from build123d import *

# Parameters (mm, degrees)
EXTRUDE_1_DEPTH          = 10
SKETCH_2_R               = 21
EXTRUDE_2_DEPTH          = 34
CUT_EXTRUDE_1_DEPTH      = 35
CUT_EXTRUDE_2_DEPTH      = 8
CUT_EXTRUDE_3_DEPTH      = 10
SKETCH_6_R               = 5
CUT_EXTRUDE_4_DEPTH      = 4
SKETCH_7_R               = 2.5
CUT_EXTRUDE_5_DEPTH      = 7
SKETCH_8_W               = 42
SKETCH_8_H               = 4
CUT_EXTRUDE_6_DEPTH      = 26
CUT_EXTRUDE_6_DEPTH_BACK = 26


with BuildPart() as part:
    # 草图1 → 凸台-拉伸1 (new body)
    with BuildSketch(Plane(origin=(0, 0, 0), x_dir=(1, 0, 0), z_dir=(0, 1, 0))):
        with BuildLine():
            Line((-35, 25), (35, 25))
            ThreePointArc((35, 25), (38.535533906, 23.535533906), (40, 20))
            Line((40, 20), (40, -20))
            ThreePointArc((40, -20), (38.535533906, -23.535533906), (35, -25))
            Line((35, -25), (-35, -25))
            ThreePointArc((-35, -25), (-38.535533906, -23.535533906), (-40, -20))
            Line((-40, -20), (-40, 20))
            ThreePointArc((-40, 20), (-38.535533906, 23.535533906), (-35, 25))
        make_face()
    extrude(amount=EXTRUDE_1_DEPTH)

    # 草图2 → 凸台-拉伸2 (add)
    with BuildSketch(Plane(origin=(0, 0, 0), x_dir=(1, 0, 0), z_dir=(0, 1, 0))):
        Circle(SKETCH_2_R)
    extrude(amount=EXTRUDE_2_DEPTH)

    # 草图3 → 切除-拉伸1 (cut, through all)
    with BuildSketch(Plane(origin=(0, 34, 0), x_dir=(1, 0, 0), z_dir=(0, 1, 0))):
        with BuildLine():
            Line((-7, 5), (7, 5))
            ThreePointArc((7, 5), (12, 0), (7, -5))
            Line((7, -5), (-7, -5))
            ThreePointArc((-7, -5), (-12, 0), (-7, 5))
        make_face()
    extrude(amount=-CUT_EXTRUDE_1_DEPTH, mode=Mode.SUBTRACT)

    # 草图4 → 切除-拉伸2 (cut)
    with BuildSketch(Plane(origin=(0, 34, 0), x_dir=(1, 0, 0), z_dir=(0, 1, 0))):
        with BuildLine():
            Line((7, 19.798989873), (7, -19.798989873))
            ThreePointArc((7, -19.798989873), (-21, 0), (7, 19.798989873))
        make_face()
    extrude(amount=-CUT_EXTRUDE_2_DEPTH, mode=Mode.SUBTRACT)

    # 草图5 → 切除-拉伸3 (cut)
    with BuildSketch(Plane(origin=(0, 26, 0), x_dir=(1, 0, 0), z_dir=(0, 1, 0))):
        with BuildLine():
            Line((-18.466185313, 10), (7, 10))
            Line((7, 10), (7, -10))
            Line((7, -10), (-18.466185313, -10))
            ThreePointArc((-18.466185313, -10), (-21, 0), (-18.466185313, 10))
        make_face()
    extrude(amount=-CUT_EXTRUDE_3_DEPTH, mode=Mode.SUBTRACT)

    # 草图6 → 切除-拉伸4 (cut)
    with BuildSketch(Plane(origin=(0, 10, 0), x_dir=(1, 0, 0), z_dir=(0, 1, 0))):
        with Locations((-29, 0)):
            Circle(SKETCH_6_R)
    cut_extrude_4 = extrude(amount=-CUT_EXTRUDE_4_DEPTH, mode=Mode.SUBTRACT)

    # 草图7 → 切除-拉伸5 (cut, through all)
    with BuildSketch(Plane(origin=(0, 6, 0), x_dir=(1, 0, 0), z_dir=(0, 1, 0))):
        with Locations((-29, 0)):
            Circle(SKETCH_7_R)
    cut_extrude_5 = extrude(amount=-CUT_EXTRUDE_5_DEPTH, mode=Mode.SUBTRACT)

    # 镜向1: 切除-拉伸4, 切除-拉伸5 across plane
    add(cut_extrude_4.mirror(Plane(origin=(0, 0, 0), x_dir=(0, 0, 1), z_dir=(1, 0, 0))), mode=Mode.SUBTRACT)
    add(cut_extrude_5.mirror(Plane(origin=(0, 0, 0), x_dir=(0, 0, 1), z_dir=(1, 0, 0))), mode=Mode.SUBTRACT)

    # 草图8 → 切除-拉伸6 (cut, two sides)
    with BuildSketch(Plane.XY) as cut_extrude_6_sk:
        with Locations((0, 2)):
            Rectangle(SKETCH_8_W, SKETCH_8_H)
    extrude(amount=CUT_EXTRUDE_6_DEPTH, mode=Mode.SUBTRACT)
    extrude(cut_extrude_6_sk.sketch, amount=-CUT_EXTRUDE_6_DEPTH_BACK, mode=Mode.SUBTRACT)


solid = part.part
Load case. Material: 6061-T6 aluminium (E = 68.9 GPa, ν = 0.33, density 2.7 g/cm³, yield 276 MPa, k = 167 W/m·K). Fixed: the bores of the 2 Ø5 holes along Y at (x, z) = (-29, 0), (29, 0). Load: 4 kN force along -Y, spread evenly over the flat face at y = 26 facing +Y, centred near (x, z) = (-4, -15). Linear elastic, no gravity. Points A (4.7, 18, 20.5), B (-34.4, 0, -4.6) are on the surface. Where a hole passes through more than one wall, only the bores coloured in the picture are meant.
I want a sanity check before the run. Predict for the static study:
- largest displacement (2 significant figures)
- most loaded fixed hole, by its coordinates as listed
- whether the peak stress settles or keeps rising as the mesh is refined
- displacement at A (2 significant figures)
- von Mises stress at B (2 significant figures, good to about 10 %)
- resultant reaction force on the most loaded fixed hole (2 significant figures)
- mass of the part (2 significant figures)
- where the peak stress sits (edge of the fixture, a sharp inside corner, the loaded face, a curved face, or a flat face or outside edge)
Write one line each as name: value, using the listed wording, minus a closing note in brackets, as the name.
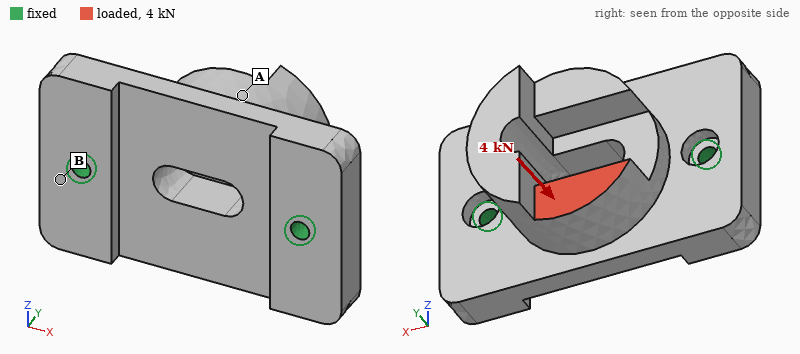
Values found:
largest displacement: 0.16 mm
most loaded fixed hole, by its coordinates as listed: (-29, 0)
whether the peak stress settles or keeps rising as the mesh is refined: keeps rising
displacement at A: 0.081 mm
von Mises stress at B: 55 MPa
resultant reaction force on the most loaded fixed hole: 3.1 kN
mass of the part: 130 g
where the peak stress sits: edge of the fixture
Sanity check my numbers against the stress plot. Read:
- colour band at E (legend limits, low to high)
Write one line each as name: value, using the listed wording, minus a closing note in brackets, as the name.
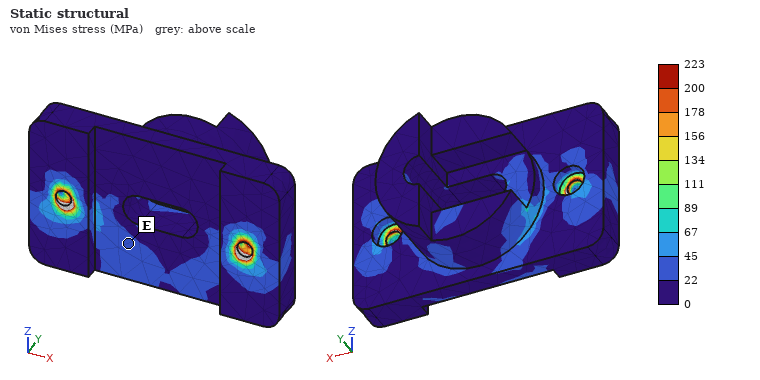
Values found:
colour band at E: 22 to 45 MPa
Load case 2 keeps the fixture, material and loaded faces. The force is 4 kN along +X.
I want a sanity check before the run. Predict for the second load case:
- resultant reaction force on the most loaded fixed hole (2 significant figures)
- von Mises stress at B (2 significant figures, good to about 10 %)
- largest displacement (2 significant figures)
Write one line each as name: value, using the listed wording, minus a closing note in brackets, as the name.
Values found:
resultant reaction force on the most loaded fixed hole: 2.9 kN
von Mises stress at B: 18 MPa
largest displacement: 41 µm
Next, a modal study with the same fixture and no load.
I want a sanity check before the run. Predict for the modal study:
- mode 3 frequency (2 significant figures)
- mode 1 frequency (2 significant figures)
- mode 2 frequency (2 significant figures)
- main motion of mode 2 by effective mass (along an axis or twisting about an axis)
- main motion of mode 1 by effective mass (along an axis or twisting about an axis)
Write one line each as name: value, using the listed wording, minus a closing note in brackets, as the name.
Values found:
mode 3 frequency: 9300 Hz
mode 1 frequency: 3300 Hz
mode 2 frequency: 8300 Hz
main motion of mode 2 by effective mass: along Y
main motion of mode 1 by effective mass: along Z
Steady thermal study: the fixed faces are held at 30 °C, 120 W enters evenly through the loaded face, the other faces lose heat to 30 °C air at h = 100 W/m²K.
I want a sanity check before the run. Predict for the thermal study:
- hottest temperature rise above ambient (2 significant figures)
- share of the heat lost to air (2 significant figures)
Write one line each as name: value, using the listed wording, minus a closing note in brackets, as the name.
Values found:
hottest temperature rise above ambient: 74 K
share of the heat lost to air: 22 %
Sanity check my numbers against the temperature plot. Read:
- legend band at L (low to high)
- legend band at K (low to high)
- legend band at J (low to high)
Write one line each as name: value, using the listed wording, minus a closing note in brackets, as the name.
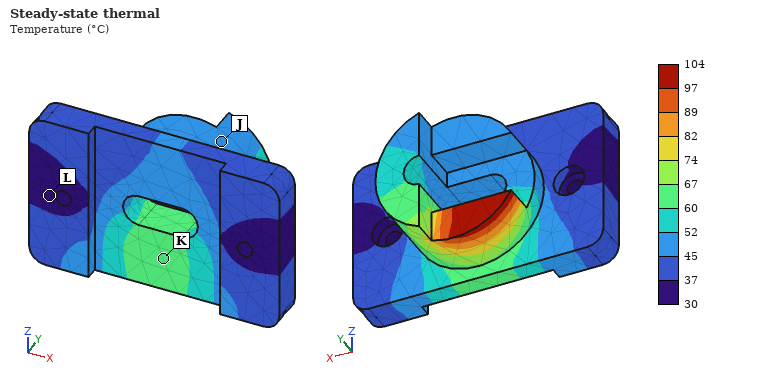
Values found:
legend band at L: 30 to 37 °C
legend band at K: 60 to 67 °C
legend band at J: 45 to 52 °C
